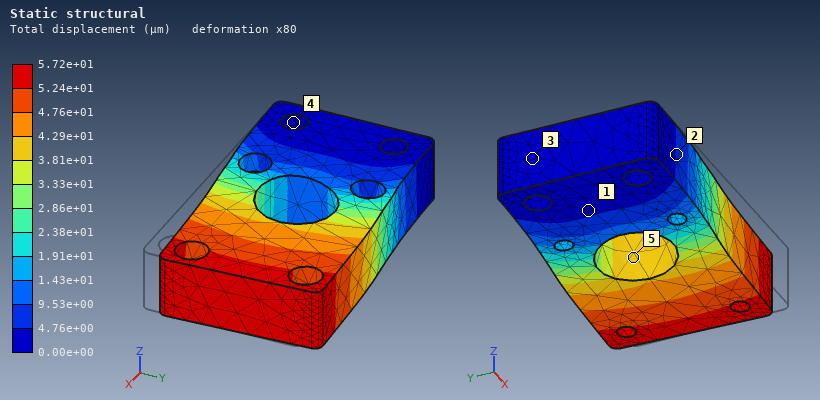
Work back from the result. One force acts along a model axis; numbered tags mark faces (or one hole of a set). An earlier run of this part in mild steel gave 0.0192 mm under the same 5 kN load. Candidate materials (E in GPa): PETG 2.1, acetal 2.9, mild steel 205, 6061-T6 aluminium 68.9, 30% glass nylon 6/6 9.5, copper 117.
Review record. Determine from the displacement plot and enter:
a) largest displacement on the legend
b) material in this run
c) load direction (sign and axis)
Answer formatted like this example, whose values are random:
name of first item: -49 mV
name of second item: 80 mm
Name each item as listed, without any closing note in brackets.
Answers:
largest displacement on the legend: 5.72e+01 µm
material in this run: 6061-T6 aluminium
load direction: +Y
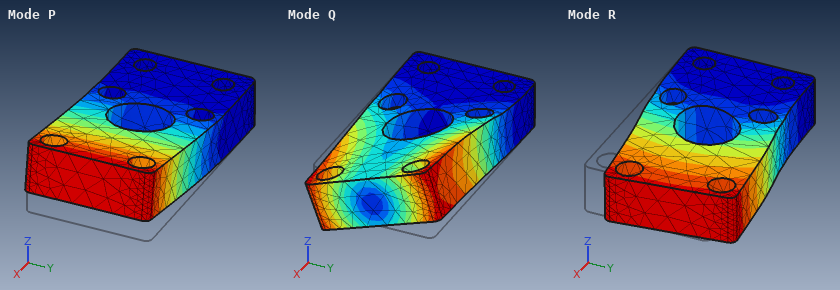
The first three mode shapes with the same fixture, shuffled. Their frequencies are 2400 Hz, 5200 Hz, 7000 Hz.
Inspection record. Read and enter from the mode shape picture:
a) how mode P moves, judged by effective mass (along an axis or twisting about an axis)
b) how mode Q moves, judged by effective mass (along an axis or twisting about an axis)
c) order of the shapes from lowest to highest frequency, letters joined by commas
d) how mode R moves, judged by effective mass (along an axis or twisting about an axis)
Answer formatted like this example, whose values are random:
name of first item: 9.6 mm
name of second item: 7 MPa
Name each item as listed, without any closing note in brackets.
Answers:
how mode P moves, judged by effective mass: along Z
how mode Q moves, judged by effective mass: twisting about X
order of the shapes from lowest to highest frequency, letters joined by commas: P, R, Q
how mode R moves, judged by effective mass: along Y
